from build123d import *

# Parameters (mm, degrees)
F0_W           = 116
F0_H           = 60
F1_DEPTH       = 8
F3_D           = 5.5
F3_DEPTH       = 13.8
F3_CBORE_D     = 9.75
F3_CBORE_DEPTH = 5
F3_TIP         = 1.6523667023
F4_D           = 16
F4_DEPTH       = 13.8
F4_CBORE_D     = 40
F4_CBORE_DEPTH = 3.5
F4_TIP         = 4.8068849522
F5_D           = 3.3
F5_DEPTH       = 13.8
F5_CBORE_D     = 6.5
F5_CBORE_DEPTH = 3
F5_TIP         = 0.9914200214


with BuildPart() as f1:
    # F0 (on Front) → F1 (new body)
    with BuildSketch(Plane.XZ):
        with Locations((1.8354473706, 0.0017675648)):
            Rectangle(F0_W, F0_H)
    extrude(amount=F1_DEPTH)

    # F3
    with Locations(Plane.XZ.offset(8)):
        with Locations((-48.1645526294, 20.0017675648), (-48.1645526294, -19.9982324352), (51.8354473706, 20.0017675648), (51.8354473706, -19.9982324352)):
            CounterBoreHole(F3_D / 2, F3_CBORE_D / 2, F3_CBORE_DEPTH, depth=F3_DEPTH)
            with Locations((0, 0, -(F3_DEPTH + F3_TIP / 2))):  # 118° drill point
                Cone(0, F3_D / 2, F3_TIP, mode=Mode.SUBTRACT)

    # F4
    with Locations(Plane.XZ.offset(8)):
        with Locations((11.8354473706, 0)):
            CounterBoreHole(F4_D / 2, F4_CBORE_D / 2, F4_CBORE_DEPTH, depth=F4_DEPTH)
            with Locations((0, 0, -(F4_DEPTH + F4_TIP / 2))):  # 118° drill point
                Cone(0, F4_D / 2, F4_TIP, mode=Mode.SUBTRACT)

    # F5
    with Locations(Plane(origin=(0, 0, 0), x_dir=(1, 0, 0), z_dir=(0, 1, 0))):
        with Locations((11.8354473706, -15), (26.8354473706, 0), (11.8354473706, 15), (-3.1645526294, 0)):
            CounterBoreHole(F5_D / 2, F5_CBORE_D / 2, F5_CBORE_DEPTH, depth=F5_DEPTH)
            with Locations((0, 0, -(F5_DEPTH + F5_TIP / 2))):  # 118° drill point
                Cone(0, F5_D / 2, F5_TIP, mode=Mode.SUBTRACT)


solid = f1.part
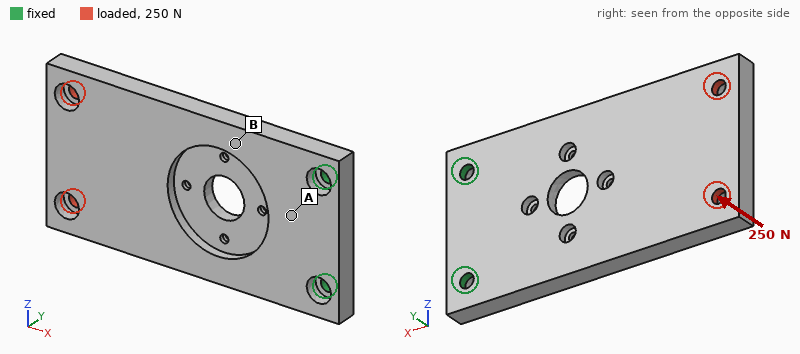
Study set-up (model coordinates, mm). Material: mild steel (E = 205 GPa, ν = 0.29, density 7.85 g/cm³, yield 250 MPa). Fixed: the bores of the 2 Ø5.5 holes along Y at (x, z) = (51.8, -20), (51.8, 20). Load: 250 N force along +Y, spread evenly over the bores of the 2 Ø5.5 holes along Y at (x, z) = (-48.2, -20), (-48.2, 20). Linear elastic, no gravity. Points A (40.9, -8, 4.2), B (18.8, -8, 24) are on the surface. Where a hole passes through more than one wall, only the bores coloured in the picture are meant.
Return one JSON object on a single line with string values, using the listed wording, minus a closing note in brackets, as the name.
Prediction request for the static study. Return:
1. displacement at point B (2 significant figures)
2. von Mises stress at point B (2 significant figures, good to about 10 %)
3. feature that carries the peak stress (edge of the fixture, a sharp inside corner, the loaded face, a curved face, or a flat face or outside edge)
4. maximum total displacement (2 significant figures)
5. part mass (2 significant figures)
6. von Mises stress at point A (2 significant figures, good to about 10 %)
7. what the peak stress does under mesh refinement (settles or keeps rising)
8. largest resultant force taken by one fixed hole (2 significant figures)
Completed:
{"displacement at point B": "0.068 mm", "von Mises stress at point B": "57 MPa", "feature that carries the peak stress": "edge of the fixture", "maximum total displacement": "0.39 mm", "part mass": "380 g", "von Mises stress at point A": "27 MPa", "what the peak stress does under mesh refinement": "keeps rising", "largest resultant force taken by one fixed hole": "280 N"}
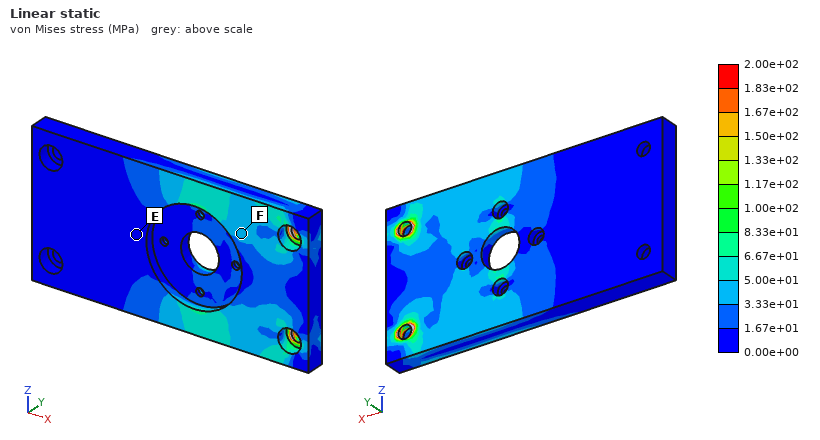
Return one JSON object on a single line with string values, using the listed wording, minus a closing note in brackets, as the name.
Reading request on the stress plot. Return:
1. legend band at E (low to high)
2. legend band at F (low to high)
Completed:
{"legend band at E": "0.00e+00 to 1.67e+01 MPa", "legend band at F": "3.33e+01 to 5.00e+01 MPa"}
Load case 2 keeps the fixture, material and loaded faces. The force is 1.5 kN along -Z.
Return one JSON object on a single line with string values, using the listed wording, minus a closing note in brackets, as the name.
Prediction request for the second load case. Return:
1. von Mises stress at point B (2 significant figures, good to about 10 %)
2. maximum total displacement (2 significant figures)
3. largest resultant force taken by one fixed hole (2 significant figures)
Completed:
{"von Mises stress at point B": "17 MPa", "maximum total displacement": "52 µm", "largest resultant force taken by one fixed hole": "3.6 kN"}
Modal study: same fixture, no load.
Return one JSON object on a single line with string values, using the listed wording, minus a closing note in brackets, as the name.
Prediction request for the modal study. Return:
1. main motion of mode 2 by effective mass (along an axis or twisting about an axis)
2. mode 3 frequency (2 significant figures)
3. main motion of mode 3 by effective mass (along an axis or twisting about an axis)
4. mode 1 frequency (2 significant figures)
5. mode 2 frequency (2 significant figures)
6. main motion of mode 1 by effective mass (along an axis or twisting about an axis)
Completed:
{"main motion of mode 2 by effective mass": "twisting about X", "mode 3 frequency": "2600 Hz", "main motion of mode 3 by effective mass": "along Z", "mode 1 frequency": "380 Hz", "mode 2 frequency": "1700 Hz", "main motion of mode 1 by effective mass": "along Y"}
